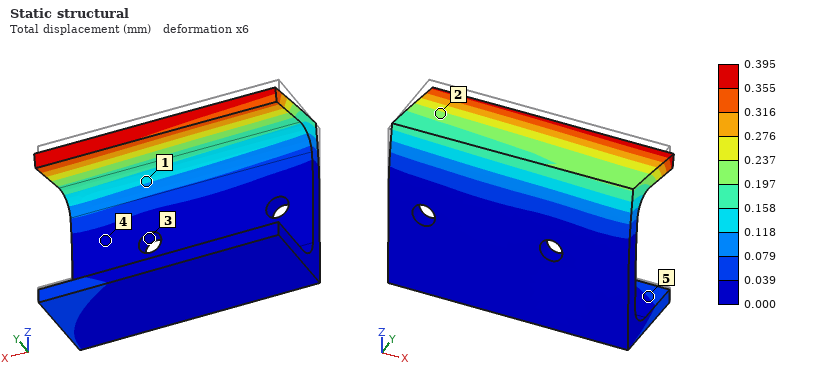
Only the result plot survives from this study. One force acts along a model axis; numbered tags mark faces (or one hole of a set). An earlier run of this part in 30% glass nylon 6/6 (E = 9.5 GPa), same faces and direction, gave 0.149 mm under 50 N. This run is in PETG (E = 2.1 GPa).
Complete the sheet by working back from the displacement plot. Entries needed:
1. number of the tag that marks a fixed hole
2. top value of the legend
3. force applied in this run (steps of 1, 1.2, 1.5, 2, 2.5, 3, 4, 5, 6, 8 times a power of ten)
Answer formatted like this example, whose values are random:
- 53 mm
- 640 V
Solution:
- 3
- 0.395 mm
- 30 N
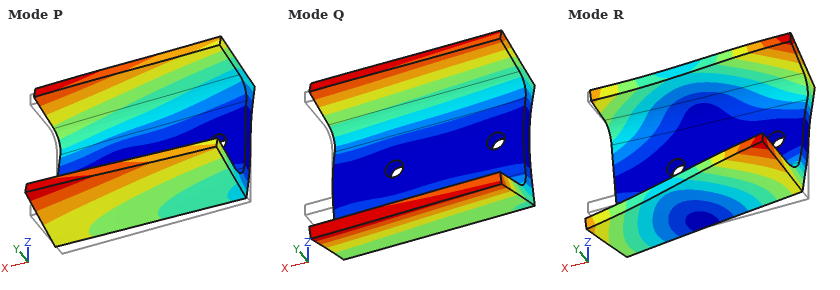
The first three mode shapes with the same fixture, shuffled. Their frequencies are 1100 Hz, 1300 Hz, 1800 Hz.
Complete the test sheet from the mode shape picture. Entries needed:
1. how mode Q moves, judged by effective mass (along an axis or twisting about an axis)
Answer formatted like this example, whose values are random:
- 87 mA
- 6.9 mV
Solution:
- along Y
